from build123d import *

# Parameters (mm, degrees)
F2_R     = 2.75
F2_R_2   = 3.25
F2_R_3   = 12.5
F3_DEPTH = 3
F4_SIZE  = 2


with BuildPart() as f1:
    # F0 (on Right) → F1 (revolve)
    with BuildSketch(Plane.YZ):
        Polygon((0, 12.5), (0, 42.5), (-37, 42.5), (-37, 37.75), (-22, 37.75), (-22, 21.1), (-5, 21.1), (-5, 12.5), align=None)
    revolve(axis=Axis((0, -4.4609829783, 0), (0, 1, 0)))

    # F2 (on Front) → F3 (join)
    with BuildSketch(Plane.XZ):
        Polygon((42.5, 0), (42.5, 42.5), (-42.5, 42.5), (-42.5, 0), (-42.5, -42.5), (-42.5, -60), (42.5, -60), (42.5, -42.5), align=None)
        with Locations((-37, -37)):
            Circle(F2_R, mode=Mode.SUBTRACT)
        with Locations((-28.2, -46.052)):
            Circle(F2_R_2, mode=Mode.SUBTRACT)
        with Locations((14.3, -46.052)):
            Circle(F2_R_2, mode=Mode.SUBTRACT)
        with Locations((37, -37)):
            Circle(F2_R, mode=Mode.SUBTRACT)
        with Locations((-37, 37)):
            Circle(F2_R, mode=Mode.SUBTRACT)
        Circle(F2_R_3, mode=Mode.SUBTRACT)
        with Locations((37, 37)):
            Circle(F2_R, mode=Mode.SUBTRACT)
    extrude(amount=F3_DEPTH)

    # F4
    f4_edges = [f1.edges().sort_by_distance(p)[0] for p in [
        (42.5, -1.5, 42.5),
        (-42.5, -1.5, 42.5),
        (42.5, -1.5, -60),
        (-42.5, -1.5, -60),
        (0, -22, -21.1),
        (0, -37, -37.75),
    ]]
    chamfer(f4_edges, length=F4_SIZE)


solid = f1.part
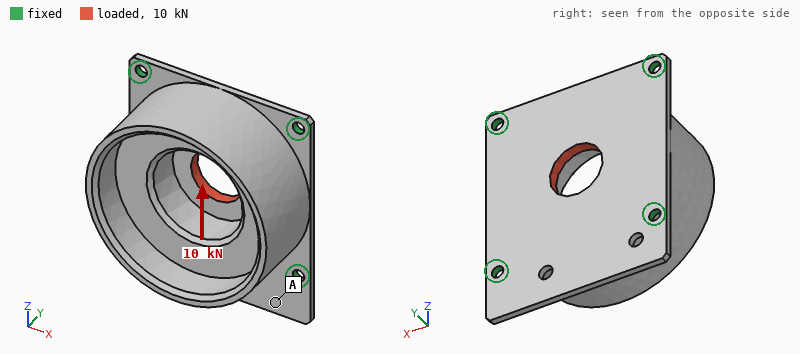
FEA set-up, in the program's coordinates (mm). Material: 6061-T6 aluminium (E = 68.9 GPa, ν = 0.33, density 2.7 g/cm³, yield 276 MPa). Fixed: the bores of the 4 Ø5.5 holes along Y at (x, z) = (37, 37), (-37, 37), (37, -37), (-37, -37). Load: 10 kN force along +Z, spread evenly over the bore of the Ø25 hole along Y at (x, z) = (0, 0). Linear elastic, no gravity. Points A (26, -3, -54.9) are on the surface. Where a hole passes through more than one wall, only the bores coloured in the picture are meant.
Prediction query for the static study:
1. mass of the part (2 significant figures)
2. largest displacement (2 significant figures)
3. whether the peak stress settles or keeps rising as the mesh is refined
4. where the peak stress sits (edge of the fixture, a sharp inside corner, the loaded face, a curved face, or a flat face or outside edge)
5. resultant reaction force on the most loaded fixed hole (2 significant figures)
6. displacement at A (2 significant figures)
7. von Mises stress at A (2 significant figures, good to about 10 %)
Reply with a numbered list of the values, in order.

1. 340 g
2. 23 µm
3. keeps rising
4. edge of the fixture
5. 2.7 kN
6. 9.8 µm
7. 11 MPa
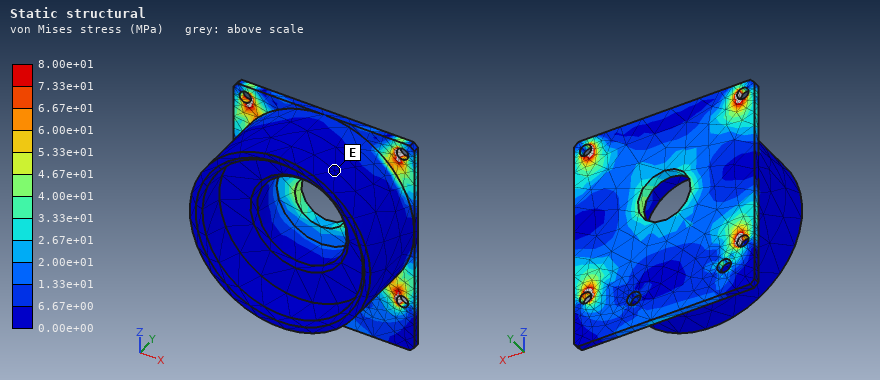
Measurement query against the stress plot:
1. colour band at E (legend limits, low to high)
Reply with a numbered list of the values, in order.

1. 0.00e+00 to 6.67e+00 MPa
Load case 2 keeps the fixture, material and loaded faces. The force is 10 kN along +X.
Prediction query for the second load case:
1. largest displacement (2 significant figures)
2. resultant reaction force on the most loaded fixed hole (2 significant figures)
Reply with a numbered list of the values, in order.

1. 23 µm
2. 2.7 kN
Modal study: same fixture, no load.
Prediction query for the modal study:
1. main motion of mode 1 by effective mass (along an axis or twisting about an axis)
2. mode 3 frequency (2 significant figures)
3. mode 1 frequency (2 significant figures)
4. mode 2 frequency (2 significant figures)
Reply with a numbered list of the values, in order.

1. along Y
2. 3400 Hz
3. 2900 Hz
4. 3300 Hz
